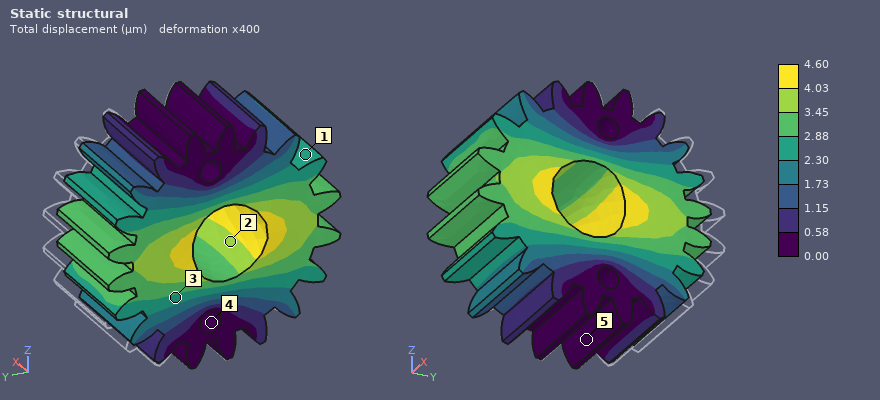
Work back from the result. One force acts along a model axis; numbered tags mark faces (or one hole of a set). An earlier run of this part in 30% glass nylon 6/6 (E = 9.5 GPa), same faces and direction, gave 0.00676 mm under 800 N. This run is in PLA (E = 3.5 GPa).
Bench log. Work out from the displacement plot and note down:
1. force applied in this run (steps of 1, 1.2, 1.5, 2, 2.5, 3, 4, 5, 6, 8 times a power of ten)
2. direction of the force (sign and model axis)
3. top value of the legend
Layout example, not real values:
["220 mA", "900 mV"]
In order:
["200 N", "-Y", "4.60 µm"]
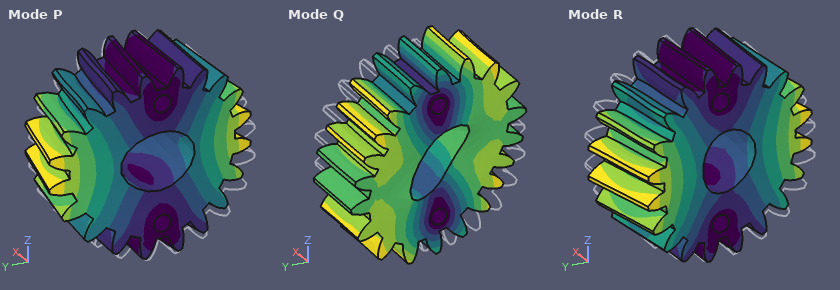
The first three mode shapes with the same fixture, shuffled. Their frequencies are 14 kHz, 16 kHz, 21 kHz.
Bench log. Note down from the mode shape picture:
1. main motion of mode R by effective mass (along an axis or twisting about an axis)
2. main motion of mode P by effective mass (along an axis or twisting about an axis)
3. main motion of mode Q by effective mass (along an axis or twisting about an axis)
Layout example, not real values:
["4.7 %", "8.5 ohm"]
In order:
["twisting about Z", "along X", "twisting about X"]
